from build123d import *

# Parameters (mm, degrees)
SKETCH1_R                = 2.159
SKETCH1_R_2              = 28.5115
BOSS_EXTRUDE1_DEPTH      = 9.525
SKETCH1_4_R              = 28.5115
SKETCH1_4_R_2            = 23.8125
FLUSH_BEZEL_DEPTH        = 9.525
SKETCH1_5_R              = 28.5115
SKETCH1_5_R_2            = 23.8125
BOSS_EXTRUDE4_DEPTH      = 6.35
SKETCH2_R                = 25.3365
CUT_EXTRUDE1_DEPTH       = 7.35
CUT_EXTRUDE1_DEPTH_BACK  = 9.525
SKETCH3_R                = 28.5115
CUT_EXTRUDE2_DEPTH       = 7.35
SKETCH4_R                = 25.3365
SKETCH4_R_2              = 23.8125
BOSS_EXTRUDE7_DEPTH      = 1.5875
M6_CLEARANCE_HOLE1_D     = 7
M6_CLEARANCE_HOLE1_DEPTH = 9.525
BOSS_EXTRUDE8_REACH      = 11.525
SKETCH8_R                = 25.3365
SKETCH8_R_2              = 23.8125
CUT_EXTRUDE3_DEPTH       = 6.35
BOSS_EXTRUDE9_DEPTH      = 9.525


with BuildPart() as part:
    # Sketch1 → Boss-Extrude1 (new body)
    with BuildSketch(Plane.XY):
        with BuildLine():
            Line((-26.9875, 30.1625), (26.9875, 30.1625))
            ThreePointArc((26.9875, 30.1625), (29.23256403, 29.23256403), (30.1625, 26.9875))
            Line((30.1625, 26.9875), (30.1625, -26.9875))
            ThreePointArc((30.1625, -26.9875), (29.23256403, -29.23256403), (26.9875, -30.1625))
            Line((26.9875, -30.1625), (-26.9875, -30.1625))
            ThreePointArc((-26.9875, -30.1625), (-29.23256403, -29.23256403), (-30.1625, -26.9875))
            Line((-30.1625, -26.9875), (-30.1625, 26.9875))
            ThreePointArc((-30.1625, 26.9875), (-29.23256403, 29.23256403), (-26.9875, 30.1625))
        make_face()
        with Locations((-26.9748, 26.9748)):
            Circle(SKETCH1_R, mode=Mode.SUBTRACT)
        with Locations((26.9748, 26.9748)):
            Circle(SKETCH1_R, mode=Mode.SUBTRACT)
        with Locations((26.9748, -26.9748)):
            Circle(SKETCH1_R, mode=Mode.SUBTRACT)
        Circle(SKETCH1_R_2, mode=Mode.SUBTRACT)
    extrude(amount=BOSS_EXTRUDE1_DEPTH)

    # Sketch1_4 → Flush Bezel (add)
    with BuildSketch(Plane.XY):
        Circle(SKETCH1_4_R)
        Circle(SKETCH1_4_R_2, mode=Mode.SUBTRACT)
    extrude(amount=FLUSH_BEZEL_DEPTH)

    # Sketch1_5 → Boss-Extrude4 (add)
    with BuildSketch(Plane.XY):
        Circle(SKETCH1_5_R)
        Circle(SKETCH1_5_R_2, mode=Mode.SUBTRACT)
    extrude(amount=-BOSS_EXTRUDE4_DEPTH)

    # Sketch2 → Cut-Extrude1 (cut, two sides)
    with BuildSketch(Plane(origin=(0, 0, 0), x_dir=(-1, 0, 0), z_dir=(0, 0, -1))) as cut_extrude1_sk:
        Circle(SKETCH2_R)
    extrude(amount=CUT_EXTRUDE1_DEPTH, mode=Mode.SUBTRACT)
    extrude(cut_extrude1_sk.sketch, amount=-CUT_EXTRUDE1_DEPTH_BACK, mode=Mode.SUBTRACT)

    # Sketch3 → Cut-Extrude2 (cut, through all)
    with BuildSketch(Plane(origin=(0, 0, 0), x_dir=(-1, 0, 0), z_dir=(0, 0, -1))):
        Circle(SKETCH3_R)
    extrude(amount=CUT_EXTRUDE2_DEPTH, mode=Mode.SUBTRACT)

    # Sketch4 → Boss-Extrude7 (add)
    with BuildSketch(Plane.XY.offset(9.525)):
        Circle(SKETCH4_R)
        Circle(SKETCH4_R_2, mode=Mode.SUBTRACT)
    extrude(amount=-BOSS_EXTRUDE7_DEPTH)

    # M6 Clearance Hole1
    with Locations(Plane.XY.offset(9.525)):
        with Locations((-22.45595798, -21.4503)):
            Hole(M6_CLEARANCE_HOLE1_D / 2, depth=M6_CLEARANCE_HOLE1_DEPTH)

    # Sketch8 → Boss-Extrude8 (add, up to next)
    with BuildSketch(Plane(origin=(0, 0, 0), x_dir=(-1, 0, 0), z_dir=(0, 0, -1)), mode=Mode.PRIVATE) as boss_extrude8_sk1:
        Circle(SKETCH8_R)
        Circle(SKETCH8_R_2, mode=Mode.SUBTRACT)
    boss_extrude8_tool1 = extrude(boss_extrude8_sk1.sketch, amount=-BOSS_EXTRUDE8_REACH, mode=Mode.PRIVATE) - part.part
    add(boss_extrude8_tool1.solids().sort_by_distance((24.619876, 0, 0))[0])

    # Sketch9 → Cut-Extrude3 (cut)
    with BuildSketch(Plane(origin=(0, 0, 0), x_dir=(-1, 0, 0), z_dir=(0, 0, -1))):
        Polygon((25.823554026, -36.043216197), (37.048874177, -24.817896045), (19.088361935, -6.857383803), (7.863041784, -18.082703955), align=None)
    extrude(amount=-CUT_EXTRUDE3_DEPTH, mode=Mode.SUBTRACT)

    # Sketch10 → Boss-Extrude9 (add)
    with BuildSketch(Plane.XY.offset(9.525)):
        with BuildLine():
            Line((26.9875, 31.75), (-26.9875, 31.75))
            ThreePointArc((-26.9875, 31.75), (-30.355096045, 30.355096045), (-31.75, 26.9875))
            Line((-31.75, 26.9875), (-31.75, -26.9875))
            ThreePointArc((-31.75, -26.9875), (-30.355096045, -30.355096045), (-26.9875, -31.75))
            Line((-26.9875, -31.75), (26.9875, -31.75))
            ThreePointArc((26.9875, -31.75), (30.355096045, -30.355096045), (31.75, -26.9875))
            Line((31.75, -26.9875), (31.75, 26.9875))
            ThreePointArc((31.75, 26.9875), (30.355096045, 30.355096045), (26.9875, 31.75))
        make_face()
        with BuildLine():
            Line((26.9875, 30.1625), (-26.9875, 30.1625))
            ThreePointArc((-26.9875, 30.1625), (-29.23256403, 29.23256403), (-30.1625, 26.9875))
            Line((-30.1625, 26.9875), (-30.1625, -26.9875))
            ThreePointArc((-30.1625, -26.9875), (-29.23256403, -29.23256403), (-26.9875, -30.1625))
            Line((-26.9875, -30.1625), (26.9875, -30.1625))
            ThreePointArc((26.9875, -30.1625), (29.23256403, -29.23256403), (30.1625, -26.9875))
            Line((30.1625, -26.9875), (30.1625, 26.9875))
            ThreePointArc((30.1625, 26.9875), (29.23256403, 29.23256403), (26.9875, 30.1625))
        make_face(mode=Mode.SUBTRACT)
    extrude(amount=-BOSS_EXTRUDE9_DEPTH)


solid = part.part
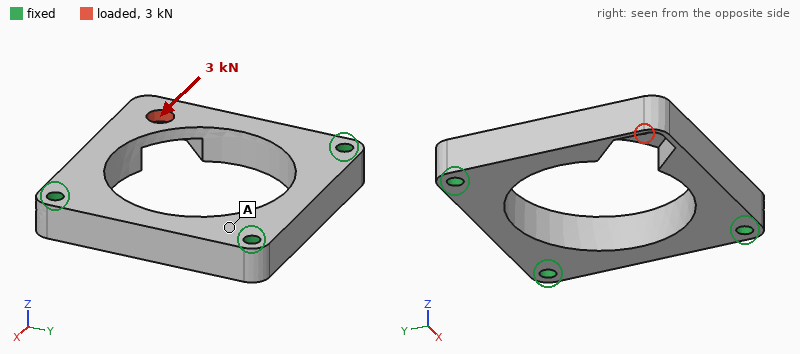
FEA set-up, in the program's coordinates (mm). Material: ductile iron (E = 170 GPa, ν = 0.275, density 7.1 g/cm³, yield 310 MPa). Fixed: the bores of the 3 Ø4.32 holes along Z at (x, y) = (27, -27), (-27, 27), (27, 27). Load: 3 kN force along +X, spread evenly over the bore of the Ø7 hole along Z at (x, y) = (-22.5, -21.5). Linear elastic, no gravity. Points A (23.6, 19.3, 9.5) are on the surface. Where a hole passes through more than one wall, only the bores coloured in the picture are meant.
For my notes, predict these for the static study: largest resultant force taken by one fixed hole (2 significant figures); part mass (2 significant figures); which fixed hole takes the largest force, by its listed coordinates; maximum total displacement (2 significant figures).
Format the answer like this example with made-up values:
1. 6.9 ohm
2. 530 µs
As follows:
1. 2.6 kN
2. 140 g
3. (27, -27)
4. 53 µm
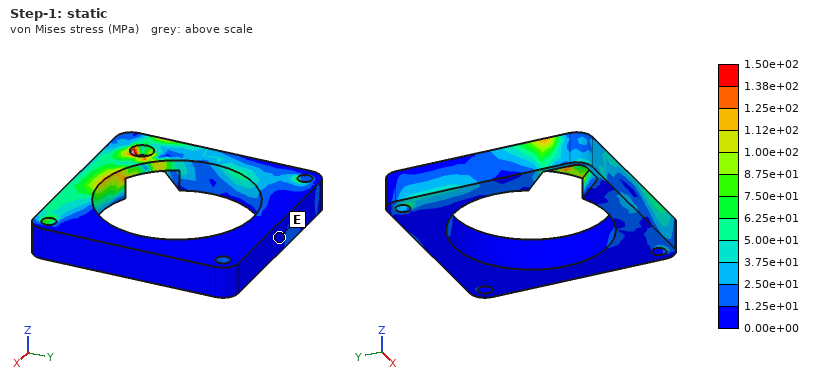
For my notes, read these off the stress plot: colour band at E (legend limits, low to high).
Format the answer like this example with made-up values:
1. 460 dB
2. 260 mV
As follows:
1. 0.00e+00 to 1.25e+01 MPa
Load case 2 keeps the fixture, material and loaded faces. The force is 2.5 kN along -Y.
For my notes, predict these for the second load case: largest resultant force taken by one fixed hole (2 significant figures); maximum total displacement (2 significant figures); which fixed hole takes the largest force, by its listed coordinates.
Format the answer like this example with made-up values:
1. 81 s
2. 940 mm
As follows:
1. 2.2 kN
2. 44 µm
3. (-27, 27)
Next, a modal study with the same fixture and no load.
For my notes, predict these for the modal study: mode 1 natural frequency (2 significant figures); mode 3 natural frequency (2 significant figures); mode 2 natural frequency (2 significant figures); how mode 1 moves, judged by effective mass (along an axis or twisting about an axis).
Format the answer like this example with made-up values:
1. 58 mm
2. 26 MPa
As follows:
1. 3600 Hz
2. 10000 Hz
3. 9100 Hz
4. along Z
